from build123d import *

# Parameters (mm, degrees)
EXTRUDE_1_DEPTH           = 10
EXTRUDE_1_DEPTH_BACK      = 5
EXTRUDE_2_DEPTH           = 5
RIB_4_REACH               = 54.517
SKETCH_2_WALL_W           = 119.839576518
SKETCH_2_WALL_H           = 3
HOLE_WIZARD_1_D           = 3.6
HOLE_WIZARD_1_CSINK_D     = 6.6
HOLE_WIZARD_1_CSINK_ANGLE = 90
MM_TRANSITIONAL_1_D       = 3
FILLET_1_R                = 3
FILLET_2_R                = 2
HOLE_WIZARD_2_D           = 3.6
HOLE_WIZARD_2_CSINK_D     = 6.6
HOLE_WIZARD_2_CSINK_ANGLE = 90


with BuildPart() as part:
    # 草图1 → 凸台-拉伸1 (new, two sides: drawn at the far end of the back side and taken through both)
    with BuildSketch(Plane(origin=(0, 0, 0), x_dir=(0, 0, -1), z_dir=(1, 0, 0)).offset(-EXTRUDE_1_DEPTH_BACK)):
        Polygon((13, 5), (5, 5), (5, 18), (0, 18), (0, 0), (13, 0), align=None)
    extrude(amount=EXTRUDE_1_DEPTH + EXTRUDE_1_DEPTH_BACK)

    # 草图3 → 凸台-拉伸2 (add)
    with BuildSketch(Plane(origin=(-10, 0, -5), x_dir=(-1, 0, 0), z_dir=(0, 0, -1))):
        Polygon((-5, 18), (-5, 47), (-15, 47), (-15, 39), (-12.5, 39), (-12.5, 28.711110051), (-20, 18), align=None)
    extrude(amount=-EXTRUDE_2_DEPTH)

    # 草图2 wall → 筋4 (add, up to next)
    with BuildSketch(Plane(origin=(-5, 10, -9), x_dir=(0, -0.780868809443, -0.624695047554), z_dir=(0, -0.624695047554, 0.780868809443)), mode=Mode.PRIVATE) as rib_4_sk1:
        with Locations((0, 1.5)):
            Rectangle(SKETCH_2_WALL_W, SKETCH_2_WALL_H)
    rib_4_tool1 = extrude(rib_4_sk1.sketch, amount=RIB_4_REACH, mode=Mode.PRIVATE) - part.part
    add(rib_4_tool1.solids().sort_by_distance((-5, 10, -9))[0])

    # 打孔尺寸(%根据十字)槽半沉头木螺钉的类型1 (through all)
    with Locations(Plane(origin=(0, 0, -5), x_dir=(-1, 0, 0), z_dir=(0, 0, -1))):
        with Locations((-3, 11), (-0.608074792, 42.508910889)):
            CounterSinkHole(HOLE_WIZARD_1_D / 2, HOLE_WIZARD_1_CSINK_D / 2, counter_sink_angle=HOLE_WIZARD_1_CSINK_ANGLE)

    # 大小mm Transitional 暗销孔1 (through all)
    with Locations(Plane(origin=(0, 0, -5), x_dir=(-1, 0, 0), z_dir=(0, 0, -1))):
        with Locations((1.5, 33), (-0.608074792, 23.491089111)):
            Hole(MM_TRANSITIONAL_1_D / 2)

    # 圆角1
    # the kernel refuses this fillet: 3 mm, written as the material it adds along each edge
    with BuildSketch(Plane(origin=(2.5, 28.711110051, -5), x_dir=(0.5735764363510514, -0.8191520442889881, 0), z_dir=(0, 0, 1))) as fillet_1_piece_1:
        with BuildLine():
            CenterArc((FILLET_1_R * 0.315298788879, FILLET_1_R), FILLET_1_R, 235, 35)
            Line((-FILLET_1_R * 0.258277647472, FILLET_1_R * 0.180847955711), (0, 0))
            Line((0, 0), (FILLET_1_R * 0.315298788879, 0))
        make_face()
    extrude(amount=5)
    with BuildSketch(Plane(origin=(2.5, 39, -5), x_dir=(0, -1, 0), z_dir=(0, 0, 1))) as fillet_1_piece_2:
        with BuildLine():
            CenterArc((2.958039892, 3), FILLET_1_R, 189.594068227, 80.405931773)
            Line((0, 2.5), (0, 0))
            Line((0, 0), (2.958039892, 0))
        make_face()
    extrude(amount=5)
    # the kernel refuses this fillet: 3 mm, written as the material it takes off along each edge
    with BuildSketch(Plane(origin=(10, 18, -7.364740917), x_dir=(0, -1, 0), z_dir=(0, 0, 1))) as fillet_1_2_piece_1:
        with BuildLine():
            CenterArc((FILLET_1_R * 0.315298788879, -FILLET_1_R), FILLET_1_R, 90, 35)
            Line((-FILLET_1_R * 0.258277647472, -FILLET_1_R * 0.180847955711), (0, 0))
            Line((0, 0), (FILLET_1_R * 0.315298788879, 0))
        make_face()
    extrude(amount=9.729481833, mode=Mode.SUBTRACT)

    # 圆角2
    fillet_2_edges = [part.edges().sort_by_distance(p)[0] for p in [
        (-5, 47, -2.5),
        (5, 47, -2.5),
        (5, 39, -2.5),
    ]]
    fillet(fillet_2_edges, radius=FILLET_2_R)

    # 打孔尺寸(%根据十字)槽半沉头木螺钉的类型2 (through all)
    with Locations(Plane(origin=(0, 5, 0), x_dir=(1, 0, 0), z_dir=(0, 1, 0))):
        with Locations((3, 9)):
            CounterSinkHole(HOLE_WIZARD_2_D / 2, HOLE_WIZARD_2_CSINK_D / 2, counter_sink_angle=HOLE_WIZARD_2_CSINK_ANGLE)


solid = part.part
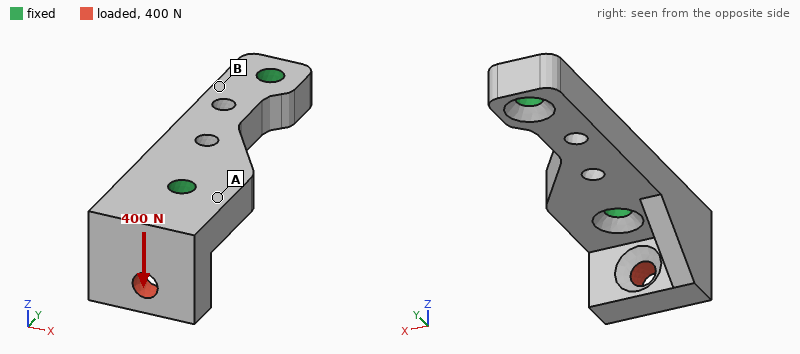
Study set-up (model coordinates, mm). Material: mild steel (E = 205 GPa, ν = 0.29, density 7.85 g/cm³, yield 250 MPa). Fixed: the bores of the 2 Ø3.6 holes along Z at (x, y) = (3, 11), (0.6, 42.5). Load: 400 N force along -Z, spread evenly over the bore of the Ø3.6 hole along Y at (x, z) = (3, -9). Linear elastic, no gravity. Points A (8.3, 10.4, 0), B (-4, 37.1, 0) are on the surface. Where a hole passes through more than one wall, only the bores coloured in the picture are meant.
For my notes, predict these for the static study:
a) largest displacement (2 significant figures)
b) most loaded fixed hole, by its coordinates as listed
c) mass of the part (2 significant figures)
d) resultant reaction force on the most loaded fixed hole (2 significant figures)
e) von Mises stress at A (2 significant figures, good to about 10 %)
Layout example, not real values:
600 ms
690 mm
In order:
8.9 µm
(3, 11)
25 g
430 N
22 MPa
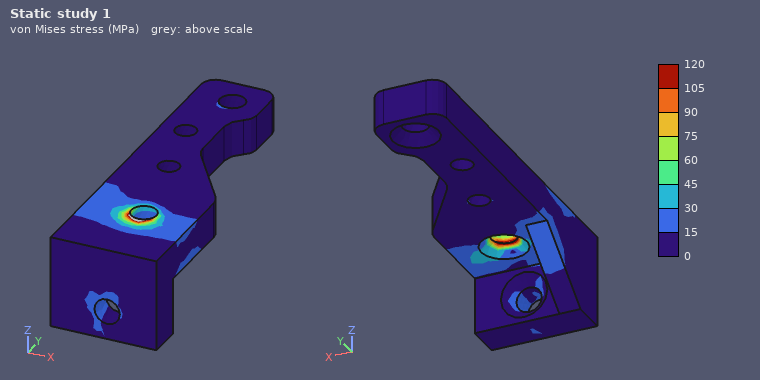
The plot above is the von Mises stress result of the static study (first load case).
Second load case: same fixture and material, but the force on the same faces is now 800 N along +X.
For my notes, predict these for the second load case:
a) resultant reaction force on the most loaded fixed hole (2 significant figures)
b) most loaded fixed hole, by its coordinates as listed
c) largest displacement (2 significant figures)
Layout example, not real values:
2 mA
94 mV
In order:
930 N
(3, 11)
19 µm
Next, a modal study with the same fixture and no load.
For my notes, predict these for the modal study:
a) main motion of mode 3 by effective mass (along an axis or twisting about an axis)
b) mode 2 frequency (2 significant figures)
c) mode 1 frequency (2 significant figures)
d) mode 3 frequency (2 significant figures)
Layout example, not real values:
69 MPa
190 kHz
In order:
along Z
16 kHz
14 kHz
23 kHz
